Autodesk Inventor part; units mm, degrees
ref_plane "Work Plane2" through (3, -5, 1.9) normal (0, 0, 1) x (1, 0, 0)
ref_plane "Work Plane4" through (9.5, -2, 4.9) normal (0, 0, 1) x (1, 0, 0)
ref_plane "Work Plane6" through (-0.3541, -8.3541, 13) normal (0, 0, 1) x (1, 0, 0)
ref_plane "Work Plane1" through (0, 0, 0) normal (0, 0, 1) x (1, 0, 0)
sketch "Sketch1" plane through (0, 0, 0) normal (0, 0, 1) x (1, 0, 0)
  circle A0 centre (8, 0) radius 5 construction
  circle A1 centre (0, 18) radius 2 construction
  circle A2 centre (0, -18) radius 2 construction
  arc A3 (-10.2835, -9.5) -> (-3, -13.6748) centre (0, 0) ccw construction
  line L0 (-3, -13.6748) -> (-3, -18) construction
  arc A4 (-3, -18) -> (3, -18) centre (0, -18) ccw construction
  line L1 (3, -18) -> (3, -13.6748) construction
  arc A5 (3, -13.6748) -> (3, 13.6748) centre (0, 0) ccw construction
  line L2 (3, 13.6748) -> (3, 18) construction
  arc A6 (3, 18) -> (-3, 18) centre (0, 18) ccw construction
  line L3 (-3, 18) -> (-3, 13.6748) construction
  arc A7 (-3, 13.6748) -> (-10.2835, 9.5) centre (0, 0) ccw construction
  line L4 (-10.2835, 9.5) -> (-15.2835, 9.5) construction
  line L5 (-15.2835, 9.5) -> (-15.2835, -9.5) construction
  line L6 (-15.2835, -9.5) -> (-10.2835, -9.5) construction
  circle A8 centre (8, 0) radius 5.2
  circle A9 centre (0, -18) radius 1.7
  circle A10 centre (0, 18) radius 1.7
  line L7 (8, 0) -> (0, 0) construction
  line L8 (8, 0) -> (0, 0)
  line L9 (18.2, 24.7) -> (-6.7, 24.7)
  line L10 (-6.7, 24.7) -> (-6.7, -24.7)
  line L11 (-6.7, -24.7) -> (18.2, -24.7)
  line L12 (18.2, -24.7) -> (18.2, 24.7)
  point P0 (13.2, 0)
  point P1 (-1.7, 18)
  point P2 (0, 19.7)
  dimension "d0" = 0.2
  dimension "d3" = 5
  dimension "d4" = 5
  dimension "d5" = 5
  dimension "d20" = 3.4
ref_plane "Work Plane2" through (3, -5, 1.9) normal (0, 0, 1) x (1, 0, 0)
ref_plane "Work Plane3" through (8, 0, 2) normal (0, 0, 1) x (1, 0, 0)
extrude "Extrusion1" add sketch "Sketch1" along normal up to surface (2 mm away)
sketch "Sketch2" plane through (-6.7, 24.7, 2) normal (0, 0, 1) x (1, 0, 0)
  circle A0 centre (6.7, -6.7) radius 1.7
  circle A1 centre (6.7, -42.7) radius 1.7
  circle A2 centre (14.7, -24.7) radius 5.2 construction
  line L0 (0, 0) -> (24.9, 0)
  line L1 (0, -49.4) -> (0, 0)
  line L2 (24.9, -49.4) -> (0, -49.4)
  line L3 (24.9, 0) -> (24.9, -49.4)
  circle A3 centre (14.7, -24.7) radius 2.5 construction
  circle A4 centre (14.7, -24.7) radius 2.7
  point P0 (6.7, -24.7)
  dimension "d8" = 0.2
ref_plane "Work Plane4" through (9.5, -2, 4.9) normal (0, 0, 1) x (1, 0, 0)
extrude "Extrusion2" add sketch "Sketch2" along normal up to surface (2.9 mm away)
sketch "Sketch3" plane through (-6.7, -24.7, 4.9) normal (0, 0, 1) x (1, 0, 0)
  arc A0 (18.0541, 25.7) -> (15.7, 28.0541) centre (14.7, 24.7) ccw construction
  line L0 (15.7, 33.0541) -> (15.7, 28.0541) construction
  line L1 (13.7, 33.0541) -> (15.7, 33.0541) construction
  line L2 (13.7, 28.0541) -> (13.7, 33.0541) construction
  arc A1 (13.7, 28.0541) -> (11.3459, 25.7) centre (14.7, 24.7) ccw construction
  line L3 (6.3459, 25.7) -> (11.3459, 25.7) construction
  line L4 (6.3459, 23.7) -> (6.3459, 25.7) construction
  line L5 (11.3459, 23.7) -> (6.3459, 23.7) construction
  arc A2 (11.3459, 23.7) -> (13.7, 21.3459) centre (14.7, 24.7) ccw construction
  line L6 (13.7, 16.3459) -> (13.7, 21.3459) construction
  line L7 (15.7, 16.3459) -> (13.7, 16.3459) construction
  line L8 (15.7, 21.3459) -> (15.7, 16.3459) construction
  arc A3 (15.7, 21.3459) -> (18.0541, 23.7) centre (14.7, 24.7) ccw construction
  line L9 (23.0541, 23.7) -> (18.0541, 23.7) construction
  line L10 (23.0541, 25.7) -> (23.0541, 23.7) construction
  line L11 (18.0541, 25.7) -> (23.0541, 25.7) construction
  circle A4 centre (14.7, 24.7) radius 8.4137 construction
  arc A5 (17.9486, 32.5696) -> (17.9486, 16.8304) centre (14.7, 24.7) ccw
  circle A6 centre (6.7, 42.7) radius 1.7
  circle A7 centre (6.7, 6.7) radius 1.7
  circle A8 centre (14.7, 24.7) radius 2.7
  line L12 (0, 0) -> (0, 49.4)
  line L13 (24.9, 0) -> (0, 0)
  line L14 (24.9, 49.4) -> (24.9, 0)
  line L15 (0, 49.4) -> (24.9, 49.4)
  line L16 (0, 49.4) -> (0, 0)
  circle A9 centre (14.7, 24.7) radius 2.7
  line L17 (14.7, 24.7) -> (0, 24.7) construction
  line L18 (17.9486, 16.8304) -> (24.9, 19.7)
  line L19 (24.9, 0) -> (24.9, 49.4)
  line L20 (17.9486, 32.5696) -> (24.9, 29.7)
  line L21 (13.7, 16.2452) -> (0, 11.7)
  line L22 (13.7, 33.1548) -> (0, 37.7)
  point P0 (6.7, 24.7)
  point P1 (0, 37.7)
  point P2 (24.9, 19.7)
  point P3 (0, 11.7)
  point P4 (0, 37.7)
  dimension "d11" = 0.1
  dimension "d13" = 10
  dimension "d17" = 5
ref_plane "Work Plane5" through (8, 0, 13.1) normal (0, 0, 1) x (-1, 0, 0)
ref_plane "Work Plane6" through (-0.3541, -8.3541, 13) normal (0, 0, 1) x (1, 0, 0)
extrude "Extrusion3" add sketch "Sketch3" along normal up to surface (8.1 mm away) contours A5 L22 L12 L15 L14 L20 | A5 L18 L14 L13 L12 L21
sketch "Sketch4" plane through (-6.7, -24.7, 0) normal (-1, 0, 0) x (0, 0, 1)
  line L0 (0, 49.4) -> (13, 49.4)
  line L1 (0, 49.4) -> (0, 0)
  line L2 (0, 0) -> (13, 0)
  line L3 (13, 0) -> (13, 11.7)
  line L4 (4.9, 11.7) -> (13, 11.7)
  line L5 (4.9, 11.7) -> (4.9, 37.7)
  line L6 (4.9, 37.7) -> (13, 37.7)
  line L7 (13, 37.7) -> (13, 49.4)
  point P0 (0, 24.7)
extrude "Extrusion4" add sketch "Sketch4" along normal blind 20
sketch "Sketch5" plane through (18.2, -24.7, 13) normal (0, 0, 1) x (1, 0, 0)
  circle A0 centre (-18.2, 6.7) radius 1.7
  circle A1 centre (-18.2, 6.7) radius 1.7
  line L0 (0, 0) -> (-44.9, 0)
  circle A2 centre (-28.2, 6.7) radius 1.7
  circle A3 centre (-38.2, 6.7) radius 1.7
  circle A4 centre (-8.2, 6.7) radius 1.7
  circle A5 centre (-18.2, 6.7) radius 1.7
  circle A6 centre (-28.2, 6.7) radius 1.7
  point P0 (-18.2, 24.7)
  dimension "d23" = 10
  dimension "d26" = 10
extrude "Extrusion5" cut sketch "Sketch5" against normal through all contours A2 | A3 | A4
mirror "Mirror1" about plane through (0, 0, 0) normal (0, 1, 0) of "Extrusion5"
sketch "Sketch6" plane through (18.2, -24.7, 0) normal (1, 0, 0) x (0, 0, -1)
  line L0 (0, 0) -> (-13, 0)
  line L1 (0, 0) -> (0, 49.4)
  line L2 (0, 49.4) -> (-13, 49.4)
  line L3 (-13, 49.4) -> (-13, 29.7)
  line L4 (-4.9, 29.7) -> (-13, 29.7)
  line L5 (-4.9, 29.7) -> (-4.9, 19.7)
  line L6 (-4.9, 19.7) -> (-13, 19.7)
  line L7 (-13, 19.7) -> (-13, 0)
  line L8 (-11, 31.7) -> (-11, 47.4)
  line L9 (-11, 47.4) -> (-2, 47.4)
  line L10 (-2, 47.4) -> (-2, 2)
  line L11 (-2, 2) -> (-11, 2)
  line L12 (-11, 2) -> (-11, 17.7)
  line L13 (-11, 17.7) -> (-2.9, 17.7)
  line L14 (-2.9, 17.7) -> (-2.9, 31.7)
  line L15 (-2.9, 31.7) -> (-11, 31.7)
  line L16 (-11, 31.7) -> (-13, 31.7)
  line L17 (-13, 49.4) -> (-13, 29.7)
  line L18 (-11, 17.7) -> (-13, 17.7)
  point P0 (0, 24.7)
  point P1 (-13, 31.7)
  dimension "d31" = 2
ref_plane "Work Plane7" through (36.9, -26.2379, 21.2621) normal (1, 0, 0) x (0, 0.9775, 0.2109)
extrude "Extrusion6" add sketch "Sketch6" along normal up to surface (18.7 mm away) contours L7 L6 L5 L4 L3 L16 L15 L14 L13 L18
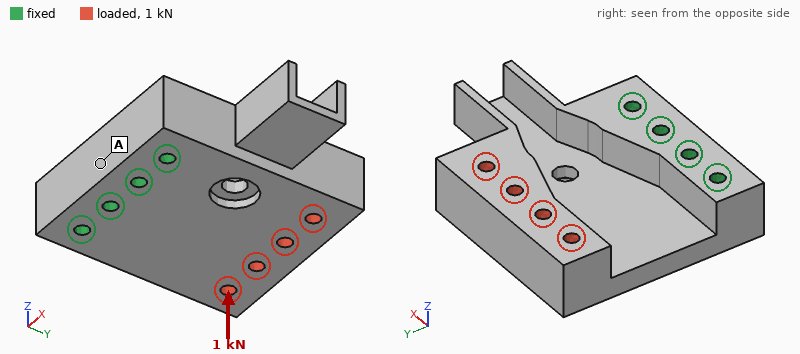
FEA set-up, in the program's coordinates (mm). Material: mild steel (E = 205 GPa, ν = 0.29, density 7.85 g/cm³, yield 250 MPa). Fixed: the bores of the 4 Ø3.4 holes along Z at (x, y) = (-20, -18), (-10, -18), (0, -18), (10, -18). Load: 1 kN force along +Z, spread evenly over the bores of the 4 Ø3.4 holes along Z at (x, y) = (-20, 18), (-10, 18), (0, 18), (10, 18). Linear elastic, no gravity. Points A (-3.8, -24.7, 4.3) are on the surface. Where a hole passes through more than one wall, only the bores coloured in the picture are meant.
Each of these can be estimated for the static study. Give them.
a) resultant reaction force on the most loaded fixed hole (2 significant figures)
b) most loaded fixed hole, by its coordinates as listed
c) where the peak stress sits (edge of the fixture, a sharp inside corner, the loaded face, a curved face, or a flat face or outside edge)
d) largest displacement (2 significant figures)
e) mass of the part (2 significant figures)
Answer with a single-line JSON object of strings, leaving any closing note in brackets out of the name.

{"resultant reaction force on the most loaded fixed hole": "400 N", "most loaded fixed hole, by its coordinates as listed": "(0, -18)", "where the peak stress sits": "a curved face", "largest displacement": "0.17 mm", "mass of the part": "160 g"}
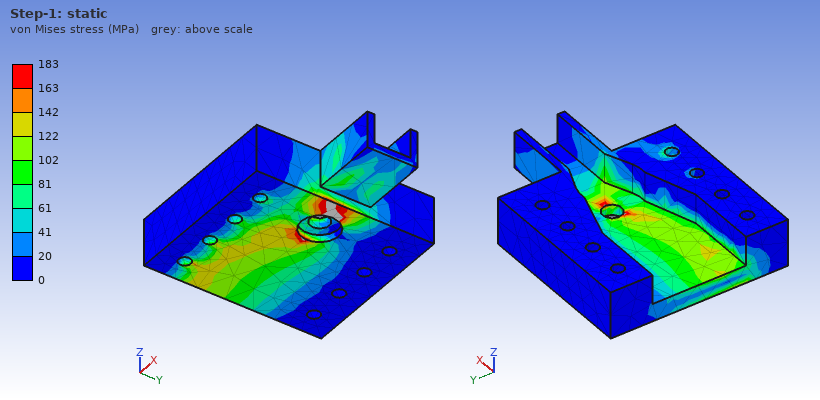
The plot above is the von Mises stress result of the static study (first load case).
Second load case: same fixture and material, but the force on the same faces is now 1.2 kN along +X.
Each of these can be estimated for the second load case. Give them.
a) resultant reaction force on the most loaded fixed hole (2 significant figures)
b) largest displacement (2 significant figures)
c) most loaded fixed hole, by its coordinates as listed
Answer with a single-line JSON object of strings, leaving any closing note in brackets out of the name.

{"resultant reaction force on the most loaded fixed hole": "1.4 kN", "largest displacement": "14 µm", "most loaded fixed hole, by its coordinates as listed": "(10, -18)"}
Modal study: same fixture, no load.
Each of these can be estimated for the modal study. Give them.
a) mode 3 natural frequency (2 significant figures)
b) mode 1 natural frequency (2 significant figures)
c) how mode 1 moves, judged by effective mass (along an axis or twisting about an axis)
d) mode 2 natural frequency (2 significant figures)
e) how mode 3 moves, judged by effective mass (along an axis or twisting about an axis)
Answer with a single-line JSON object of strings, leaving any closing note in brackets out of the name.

{"mode 3 natural frequency": "8400 Hz", "mode 1 natural frequency": "1800 Hz", "how mode 1 moves, judged by effective mass": "along Z", "mode 2 natural frequency": "4600 Hz", "how mode 3 moves, judged by effective mass": "along X"}
